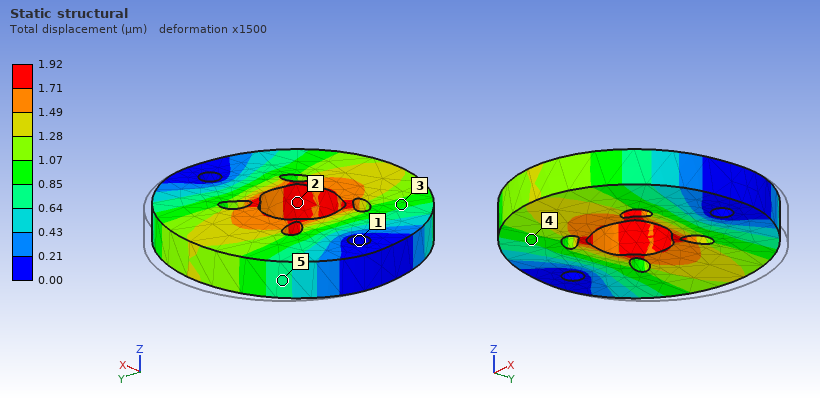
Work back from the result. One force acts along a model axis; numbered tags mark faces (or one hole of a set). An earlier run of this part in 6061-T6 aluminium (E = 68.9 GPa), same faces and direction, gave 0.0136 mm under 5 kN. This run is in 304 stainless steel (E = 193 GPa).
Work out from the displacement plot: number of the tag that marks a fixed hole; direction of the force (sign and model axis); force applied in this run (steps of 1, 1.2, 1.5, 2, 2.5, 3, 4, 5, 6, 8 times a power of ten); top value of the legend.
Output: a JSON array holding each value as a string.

["1", "-Y", "2 kN", "1.92 µm"]
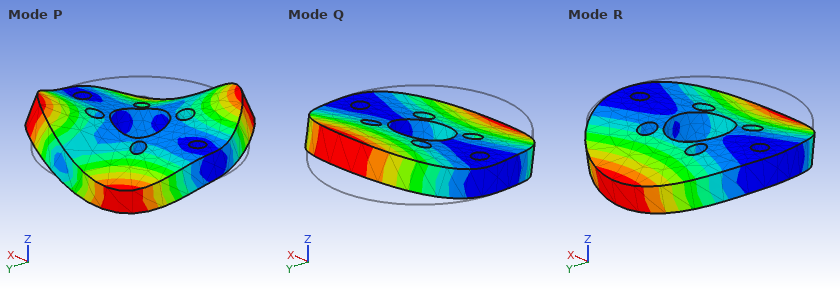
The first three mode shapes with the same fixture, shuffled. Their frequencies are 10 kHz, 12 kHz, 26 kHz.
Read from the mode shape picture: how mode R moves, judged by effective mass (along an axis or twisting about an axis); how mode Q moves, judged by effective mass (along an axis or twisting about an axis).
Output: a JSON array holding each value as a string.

["along Z", "twisting about X"]
